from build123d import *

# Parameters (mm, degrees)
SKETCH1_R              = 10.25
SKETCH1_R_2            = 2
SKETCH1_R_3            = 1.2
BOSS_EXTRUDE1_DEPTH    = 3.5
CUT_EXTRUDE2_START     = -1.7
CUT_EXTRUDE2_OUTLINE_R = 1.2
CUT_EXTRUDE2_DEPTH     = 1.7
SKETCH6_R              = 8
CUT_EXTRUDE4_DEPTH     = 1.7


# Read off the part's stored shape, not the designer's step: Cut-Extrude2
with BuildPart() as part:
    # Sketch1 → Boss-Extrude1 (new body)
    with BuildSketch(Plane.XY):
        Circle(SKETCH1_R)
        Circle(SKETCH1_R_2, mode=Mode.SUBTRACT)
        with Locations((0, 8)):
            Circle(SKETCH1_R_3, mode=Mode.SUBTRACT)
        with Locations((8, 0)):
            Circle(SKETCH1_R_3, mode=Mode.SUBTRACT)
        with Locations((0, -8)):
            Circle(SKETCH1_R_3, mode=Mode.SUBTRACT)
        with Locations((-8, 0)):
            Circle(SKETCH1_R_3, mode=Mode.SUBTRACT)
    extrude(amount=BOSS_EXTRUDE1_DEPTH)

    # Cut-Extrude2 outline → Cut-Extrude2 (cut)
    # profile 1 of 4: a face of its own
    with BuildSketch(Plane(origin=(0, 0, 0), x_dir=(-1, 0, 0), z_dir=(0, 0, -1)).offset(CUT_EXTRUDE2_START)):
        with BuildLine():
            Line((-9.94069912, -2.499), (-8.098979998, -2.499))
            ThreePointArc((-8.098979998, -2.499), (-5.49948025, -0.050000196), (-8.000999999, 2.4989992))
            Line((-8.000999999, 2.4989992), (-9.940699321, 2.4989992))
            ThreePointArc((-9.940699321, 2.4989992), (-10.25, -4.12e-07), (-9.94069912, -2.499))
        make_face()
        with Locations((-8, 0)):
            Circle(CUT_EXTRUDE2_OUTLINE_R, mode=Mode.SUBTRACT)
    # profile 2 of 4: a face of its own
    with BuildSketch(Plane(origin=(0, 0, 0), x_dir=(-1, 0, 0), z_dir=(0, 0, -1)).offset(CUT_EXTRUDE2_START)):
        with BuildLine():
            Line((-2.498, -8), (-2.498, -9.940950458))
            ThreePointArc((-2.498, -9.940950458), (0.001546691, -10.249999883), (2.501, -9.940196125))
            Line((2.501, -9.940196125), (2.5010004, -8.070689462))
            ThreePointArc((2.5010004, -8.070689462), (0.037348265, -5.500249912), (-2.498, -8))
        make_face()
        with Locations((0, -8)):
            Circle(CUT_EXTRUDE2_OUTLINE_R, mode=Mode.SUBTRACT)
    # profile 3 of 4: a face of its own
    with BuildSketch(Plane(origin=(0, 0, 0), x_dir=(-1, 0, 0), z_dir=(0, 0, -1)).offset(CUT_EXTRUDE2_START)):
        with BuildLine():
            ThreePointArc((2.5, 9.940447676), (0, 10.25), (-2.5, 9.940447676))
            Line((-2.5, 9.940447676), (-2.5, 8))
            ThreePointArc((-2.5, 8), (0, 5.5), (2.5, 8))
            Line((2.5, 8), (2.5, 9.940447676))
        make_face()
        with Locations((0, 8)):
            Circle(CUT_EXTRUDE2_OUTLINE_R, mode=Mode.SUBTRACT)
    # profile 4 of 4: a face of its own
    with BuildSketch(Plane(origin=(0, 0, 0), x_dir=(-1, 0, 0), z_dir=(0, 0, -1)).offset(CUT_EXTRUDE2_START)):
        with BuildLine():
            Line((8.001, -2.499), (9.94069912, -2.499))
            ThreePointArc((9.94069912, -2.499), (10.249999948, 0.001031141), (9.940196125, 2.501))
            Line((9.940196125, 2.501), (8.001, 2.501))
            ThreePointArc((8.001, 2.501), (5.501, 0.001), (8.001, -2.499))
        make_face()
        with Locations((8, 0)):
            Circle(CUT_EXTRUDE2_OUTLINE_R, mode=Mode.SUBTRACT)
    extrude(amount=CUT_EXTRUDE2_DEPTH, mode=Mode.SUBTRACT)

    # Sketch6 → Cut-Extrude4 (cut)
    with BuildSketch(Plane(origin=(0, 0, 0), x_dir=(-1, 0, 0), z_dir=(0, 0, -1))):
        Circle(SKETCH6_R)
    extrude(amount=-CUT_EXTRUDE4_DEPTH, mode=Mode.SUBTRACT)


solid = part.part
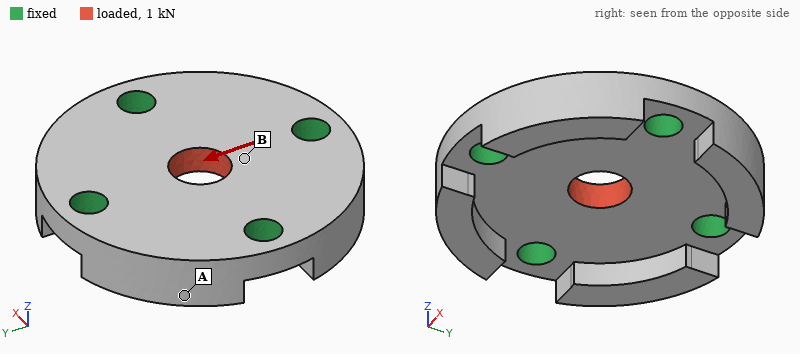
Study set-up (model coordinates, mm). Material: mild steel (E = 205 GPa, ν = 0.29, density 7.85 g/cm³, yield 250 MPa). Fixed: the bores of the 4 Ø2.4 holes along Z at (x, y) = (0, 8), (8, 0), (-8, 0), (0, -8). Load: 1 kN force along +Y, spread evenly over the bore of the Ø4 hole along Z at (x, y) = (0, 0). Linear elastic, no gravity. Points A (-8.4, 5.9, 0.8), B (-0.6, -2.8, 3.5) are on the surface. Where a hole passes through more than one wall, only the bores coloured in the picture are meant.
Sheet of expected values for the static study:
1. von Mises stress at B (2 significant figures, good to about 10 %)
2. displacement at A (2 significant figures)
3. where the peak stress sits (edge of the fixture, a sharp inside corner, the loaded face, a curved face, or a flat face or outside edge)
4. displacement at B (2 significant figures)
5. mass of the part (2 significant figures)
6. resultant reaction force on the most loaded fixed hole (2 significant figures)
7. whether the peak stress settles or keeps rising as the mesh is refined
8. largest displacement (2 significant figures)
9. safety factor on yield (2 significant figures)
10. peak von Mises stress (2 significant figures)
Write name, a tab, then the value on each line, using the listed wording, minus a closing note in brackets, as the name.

von Mises stress at B	46 MPa
displacement at A	0.33 µm
where the peak stress sits	the loaded face
displacement at B	0.89 µm
mass of the part	5.3 g
resultant reaction force on the most loaded fixed hole	330 N
whether the peak stress settles or keeps rising as the mesh is refined	settles
largest displacement	1.2 µm
safety factor on yield	3.3
peak von Mises stress	77 MPa
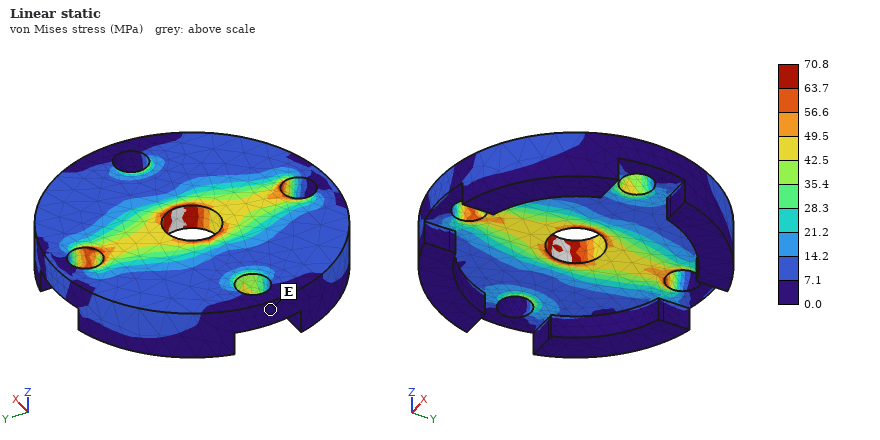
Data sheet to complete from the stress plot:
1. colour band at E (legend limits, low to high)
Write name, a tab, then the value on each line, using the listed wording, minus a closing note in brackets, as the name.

colour band at E	0.0 to 7.1 MPa
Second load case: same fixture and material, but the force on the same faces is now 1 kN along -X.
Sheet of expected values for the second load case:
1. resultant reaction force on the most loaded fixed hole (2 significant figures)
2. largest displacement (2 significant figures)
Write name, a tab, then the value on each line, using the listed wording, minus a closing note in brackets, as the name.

resultant reaction force on the most loaded fixed hole	330 N
largest displacement	1.2 µm
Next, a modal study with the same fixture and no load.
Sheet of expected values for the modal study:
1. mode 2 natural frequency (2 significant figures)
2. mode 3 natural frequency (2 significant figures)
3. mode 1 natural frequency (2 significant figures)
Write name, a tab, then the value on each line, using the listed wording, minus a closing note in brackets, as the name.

mode 2 natural frequency	51 kHz
mode 3 natural frequency	51 kHz
mode 1 natural frequency	50 kHz
